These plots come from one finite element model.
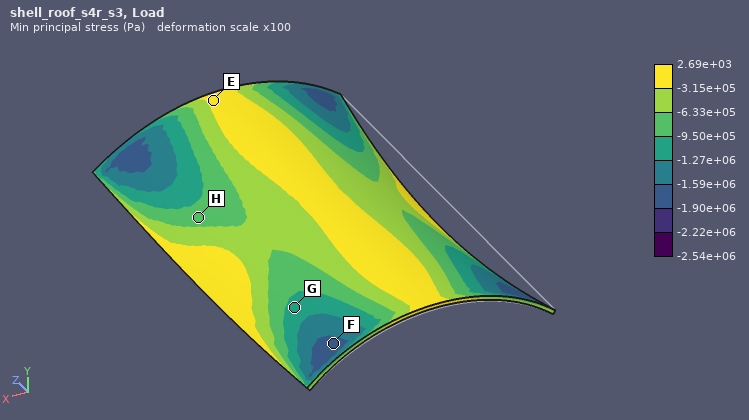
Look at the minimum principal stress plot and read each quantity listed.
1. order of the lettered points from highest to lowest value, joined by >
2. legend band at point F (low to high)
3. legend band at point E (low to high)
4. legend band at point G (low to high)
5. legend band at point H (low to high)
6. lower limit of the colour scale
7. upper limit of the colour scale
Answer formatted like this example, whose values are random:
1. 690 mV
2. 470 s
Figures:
1. E > H > G > F
2. -1.90e+06 to -1.59e+06 Pa
3. -3.15e+05 to 2.69e+03 Pa
4. -1.27e+06 to -9.50e+05 Pa
5. -9.50e+05 to -6.33e+05 Pa
6. -2.54e+06 Pa
7. 2.69e+03 Pa
